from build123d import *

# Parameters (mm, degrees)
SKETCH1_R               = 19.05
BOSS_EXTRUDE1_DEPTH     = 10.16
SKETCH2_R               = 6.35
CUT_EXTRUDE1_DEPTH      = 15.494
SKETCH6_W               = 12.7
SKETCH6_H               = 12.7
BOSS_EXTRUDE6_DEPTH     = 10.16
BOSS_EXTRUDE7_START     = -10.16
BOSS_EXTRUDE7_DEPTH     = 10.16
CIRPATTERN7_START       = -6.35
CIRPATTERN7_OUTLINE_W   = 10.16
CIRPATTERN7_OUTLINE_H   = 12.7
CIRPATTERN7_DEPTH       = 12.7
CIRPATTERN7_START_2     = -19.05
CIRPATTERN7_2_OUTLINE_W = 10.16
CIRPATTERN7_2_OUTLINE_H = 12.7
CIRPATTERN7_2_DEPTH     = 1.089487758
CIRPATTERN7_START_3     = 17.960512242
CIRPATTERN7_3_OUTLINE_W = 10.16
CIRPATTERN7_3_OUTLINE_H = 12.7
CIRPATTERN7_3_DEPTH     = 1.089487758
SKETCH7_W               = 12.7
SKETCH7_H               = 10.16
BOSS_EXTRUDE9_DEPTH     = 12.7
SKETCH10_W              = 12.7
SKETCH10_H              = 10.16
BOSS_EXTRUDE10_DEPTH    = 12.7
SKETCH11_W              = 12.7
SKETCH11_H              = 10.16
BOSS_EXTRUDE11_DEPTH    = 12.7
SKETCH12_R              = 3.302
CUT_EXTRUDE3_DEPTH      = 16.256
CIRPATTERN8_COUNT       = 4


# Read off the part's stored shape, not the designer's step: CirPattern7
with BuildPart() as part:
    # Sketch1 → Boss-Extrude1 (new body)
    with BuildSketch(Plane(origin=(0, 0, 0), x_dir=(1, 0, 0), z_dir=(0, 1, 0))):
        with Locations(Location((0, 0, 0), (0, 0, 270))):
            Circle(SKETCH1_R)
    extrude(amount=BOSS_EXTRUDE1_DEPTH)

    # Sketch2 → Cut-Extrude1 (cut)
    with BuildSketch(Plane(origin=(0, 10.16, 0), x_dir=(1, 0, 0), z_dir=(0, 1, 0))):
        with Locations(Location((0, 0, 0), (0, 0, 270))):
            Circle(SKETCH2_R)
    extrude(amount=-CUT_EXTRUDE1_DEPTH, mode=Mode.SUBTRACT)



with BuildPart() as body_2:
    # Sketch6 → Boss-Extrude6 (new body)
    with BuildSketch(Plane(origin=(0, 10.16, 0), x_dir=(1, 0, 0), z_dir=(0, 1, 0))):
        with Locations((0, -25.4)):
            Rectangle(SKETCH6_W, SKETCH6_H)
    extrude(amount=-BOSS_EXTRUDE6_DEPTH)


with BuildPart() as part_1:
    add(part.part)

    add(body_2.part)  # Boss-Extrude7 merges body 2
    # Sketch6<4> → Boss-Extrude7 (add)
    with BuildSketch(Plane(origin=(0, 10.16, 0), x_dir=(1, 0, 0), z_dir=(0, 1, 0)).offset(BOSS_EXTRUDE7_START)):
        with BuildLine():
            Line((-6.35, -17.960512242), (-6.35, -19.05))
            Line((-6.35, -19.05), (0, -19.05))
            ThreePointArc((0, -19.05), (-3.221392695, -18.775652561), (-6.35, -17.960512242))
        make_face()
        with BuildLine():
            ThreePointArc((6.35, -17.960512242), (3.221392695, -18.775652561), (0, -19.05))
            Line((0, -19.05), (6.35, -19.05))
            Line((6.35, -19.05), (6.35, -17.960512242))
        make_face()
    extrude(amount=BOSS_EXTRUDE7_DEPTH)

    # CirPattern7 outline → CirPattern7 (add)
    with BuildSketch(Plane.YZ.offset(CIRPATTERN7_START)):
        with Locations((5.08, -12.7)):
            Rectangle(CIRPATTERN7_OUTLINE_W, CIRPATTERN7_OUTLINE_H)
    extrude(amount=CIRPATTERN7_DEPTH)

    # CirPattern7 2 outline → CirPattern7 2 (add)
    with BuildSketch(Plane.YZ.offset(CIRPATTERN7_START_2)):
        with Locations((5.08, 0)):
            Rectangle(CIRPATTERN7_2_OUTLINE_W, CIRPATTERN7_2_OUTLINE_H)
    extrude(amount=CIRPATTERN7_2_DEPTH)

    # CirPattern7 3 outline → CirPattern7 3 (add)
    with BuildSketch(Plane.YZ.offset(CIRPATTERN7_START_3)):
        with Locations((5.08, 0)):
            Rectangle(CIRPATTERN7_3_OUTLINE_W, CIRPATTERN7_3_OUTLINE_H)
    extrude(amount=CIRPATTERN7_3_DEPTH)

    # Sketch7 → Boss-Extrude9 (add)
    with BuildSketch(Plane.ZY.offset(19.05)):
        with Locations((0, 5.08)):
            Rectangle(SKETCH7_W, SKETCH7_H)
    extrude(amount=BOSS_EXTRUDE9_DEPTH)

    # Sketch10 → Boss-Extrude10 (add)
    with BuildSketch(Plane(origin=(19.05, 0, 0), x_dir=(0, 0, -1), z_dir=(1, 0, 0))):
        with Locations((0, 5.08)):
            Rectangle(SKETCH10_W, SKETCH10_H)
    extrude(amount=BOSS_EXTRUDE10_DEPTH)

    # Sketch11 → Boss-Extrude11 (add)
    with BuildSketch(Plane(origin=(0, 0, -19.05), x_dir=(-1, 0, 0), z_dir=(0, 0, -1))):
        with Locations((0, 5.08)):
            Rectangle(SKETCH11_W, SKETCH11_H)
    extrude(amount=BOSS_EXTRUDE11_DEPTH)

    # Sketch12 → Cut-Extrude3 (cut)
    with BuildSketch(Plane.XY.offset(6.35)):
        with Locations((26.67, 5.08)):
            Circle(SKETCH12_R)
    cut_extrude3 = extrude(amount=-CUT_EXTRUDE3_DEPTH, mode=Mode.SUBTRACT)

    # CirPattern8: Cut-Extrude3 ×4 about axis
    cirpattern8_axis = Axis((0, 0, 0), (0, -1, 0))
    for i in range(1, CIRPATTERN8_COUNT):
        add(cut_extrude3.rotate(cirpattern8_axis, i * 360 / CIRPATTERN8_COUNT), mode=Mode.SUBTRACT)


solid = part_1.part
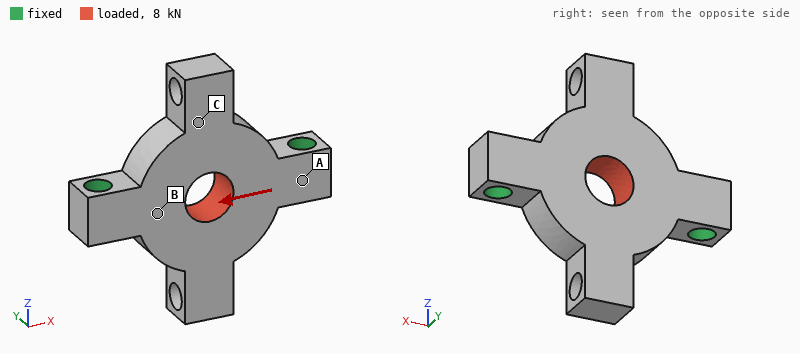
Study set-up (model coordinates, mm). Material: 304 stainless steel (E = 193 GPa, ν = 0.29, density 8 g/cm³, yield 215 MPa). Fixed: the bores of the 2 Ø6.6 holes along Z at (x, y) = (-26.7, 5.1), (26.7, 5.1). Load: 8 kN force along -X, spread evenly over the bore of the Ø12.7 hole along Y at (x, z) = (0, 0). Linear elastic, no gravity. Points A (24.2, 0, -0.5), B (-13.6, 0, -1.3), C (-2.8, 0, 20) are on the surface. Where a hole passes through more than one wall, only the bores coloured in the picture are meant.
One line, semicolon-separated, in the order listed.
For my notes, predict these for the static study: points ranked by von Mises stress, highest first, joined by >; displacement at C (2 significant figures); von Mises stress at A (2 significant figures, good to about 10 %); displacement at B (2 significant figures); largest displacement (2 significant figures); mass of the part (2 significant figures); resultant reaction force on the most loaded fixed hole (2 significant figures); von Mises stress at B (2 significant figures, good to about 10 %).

B > A > C; 1.9 µm; 15 MPa; 1.5 µm; 3.2 µm; 120 g; 4.0 kN; 28 MPa
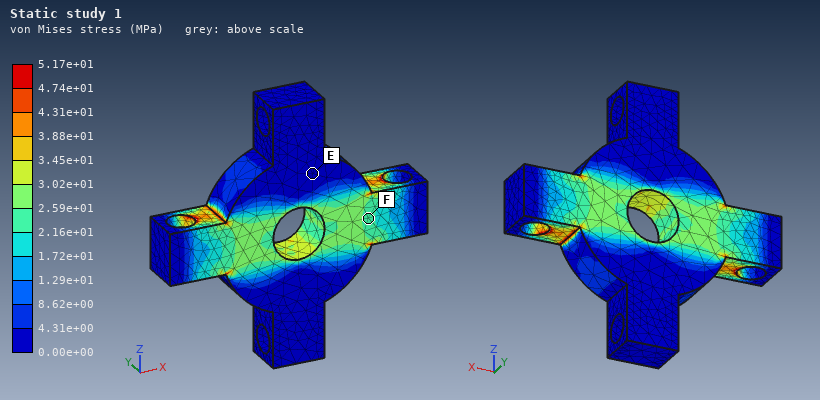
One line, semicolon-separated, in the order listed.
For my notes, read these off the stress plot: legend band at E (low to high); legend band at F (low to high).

0.00e+00 to 4.31e+00 MPa; 2.16e+01 to 2.59e+01 MPa
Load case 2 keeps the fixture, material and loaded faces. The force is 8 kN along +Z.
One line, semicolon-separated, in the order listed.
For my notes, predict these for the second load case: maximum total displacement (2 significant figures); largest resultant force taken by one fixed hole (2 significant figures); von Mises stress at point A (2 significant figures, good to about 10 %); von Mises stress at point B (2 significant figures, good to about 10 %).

8.0 µm; 4.0 kN; 27 MPa; 25 MPa
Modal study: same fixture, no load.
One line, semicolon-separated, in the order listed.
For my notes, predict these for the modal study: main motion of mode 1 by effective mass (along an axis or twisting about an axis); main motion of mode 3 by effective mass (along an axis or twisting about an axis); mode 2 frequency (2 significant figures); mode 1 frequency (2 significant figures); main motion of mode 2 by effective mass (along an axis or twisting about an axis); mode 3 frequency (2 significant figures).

twisting about X; along Z; 8000 Hz; 5800 Hz; along Y; 18 kHz
